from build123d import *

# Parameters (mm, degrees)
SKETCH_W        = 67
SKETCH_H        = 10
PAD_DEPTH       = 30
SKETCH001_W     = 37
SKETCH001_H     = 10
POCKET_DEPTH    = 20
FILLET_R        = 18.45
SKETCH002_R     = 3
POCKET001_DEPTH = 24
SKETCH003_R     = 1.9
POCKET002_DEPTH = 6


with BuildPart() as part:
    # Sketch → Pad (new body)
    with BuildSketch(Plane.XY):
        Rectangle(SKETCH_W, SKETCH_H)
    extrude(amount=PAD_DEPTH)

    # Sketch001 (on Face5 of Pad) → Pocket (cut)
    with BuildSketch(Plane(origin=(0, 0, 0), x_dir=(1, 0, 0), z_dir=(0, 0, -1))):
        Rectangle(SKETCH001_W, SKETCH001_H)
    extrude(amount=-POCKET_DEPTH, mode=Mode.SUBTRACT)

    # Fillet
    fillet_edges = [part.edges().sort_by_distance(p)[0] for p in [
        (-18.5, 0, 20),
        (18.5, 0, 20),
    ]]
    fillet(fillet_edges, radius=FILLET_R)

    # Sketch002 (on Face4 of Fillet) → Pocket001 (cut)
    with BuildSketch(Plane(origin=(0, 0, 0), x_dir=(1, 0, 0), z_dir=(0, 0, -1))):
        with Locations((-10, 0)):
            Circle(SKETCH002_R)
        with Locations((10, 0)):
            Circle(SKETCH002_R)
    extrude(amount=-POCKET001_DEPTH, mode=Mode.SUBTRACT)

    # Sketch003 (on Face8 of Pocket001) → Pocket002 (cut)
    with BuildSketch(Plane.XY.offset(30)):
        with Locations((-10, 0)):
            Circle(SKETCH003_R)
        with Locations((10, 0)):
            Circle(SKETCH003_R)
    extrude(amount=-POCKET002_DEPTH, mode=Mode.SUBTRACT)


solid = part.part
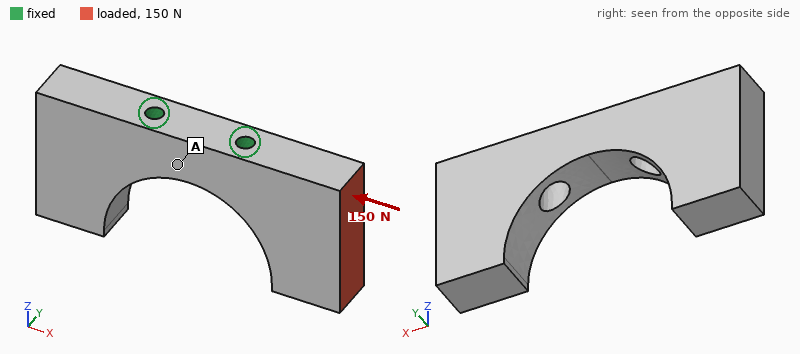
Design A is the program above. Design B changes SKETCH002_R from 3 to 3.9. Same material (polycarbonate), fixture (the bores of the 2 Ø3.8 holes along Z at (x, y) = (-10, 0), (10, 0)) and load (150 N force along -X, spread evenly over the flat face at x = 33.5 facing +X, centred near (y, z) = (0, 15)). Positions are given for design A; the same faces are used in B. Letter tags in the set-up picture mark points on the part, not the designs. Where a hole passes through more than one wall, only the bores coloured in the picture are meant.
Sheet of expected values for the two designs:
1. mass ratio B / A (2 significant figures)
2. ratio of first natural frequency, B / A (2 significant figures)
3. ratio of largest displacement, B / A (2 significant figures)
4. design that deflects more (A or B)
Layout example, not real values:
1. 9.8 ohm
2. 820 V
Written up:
1. 0.98
2. 0.95
3. 1.3
4. B
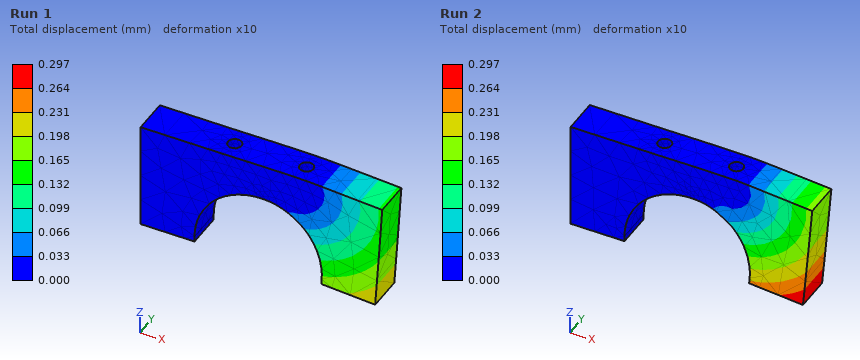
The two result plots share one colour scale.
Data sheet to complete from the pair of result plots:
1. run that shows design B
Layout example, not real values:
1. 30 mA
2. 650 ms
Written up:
1. Run 2
